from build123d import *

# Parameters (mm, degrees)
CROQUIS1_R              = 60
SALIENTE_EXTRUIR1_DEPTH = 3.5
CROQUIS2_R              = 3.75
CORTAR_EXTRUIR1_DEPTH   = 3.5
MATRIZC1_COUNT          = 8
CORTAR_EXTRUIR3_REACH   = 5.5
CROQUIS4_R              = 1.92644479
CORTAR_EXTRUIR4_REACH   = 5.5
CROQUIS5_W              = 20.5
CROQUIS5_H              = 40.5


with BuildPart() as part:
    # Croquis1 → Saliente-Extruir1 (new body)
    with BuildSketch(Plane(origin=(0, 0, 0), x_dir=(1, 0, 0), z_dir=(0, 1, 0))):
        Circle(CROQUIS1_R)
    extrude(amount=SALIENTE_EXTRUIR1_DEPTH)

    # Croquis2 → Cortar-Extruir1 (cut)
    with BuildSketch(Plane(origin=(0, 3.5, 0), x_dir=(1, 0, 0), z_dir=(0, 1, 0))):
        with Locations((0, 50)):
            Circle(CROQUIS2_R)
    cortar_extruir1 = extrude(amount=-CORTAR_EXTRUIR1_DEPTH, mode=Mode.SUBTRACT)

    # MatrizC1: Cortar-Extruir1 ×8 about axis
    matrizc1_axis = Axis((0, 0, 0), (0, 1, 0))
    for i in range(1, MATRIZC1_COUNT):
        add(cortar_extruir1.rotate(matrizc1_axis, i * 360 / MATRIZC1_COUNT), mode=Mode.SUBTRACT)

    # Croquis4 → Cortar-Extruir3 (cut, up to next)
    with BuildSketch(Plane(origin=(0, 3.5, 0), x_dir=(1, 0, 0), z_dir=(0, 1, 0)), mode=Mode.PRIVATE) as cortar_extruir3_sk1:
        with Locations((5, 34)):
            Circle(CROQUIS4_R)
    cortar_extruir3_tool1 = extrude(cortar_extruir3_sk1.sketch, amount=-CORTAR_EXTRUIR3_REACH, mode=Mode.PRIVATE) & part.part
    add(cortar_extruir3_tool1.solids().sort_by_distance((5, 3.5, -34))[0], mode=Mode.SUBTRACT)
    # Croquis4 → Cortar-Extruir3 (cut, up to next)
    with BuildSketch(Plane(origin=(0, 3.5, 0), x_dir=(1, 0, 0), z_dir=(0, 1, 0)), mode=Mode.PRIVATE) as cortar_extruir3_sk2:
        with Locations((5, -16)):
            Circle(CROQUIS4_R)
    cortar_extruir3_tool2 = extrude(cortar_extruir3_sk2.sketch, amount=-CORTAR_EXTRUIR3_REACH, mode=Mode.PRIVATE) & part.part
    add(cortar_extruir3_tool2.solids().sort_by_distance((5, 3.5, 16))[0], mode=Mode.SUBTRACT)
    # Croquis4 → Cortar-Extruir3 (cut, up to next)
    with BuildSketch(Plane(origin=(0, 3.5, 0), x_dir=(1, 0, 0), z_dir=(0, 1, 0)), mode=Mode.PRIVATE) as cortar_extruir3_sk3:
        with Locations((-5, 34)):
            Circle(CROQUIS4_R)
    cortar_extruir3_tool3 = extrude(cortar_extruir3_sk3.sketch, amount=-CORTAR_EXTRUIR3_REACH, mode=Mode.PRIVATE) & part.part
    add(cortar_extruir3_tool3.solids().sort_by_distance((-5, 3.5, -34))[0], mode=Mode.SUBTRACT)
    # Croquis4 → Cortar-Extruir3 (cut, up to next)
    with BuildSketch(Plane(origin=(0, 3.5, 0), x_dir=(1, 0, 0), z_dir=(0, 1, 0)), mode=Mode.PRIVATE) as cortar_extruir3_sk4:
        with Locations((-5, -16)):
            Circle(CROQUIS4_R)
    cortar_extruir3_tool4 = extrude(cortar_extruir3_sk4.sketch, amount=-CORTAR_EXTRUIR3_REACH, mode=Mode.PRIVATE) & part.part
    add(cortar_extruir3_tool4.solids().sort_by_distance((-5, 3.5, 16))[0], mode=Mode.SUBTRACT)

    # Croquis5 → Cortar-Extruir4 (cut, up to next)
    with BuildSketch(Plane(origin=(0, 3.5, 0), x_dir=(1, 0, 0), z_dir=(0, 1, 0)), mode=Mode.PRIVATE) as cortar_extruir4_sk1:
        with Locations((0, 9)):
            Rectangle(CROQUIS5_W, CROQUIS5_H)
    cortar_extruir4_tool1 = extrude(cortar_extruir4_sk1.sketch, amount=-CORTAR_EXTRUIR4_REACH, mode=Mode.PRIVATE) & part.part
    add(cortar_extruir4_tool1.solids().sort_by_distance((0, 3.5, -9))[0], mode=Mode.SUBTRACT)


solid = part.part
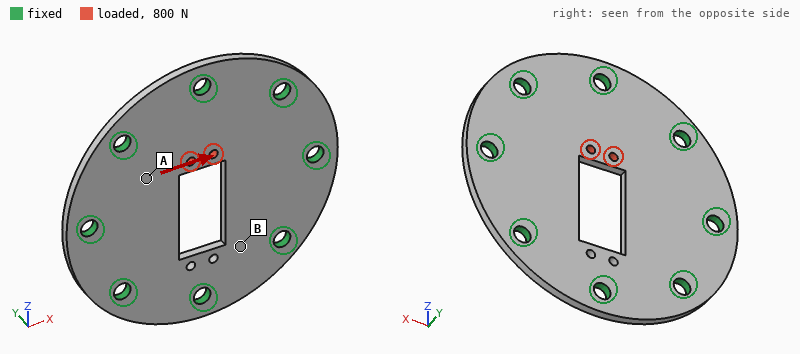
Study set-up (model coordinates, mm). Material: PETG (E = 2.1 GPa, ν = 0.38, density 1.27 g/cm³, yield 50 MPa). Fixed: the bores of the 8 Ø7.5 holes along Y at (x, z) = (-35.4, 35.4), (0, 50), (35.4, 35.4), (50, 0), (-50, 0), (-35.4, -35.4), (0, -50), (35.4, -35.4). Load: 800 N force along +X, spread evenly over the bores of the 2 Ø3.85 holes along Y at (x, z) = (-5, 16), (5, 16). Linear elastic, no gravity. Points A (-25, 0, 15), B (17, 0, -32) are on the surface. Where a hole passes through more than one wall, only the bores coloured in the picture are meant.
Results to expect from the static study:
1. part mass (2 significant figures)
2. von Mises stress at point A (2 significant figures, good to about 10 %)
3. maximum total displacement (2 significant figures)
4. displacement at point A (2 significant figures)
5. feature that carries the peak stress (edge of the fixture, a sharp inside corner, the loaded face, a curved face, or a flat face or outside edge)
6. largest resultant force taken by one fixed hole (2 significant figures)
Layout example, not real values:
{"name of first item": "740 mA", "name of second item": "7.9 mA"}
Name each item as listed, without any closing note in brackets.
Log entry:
{"part mass": "45 g", "von Mises stress at point A": "3.1 MPa", "maximum total displacement": "0.11 mm", "displacement at point A": "0.033 mm", "feature that carries the peak stress": "the loaded face", "largest resultant force taken by one fixed hole": "250 N"}
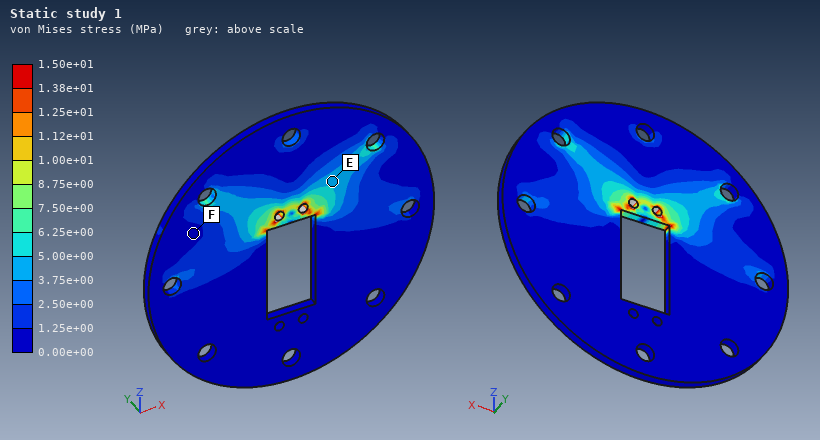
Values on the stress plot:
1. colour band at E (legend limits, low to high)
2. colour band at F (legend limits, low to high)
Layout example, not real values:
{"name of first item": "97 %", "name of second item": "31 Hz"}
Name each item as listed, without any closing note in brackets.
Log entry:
{"colour band at E": "3.75e+00 to 5.00e+00 MPa", "colour band at F": "0.00e+00 to 1.25e+00 MPa"}
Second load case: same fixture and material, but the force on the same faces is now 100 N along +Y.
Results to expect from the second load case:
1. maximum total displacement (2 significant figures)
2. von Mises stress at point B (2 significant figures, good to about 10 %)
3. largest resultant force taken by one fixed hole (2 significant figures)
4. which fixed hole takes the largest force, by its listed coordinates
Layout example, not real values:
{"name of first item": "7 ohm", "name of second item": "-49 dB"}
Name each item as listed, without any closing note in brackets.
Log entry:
{"maximum total displacement": "0.87 mm", "von Mises stress at point B": "2.2 MPa", "largest resultant force taken by one fixed hole": "31 N", "which fixed hole takes the largest force, by its listed coordinates": "(0, 50)"}
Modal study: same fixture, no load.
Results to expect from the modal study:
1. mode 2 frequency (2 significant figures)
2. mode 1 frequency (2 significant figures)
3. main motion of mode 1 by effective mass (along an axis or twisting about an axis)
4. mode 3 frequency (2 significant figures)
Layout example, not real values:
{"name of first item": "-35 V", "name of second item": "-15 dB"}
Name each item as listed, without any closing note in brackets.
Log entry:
{"mode 2 frequency": "1300 Hz", "mode 1 frequency": "960 Hz", "main motion of mode 1 by effective mass": "along Y", "mode 3 frequency": "1800 Hz"}
